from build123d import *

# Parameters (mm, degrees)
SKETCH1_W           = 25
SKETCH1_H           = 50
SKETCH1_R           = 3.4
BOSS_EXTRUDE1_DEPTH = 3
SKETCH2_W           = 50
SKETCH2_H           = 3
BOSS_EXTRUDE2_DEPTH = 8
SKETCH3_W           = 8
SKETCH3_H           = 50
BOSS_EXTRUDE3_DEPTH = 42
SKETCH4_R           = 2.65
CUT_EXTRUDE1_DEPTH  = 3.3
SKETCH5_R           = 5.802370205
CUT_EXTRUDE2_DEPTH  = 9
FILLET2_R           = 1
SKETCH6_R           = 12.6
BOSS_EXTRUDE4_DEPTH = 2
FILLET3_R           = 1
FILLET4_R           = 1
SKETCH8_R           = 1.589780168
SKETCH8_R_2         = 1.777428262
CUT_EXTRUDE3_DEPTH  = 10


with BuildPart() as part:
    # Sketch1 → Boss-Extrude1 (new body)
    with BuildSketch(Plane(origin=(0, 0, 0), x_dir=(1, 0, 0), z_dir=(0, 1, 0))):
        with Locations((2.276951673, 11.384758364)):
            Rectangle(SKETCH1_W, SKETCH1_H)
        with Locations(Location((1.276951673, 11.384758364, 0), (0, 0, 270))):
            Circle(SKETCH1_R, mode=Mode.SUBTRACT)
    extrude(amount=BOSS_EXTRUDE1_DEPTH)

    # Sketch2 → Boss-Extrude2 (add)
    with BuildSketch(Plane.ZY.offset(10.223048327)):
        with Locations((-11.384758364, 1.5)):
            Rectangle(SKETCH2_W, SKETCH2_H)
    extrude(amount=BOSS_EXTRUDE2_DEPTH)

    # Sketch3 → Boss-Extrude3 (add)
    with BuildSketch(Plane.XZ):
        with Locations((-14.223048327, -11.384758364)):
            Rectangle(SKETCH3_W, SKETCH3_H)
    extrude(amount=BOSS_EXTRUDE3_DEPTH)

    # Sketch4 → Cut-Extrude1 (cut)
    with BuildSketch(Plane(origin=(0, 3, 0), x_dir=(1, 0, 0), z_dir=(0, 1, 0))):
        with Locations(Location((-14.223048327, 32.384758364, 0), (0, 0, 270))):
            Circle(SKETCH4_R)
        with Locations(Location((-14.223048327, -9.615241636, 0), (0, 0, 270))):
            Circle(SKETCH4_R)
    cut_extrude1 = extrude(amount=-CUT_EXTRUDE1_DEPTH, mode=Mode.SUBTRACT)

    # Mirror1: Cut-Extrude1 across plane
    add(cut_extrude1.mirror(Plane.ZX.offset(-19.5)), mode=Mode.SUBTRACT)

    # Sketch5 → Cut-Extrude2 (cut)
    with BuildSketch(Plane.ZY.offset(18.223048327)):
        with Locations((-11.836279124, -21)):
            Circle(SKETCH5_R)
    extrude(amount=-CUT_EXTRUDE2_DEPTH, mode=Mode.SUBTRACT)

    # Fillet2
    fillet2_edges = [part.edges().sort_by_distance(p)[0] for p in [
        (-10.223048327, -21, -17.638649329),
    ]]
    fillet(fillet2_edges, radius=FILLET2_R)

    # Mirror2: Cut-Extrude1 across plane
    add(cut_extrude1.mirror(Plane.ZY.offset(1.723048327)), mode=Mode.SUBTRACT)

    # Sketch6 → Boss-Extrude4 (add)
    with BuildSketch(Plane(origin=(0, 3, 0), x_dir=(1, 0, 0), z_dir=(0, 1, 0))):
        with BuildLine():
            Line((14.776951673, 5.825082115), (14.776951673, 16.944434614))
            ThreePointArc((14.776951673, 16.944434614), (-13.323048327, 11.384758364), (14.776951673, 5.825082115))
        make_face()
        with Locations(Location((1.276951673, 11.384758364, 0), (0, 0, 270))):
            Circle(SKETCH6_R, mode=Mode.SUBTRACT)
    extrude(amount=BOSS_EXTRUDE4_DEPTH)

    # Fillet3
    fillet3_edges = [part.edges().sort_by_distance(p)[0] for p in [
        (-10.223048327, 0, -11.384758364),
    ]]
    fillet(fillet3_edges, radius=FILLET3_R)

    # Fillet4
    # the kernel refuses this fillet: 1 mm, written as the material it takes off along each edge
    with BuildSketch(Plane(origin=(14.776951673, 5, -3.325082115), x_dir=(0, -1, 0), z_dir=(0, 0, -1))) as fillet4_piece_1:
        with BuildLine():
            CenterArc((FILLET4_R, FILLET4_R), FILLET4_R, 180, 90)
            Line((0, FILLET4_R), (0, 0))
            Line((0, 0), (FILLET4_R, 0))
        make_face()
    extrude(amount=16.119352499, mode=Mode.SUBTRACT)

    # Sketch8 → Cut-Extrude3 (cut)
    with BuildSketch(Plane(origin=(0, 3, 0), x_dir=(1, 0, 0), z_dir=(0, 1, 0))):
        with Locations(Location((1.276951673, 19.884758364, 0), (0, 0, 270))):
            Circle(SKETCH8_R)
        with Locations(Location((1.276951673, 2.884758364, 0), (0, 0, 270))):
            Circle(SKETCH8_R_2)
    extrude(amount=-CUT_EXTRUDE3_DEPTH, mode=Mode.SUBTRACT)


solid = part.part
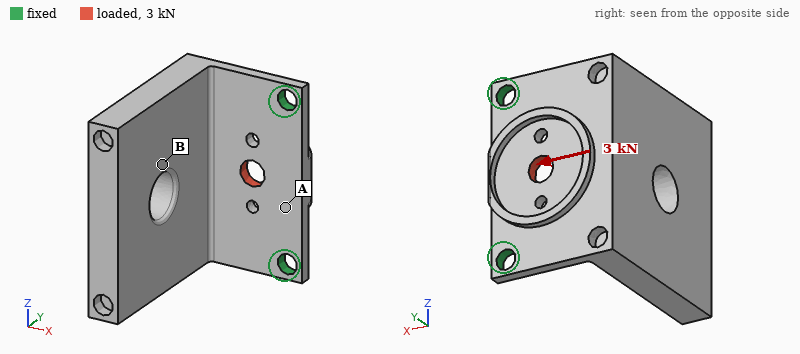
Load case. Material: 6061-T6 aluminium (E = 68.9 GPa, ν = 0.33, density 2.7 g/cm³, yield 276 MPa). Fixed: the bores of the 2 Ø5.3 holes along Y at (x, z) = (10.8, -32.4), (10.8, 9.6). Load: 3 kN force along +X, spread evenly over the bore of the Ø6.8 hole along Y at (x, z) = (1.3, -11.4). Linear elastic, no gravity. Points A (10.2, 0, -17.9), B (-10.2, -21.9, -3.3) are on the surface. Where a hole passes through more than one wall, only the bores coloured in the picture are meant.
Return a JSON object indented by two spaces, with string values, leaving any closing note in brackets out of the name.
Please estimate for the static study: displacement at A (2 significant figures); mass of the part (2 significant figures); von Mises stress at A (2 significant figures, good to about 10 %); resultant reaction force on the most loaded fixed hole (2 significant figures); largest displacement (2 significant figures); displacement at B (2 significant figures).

{
  "displacement at A": "16 µm",
  "mass of the part": "56 g",
  "von Mises stress at A": "29 MPa",
  "resultant reaction force on the most loaded fixed hole": "1.6 kN",
  "largest displacement": "31 µm",
  "displacement at B": "21 µm"
}
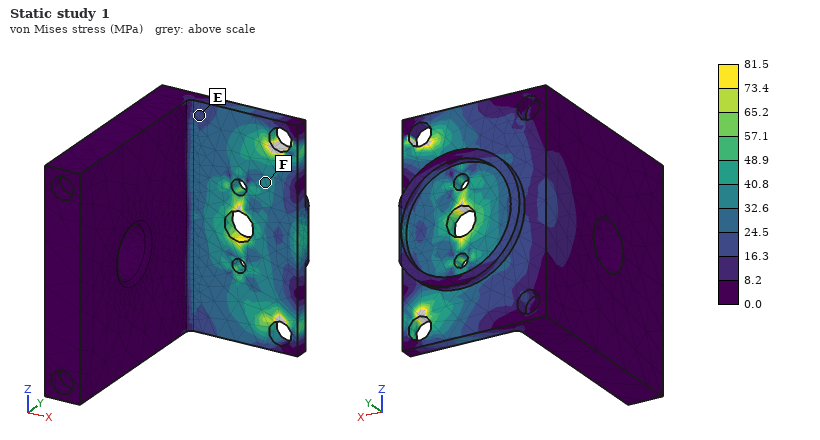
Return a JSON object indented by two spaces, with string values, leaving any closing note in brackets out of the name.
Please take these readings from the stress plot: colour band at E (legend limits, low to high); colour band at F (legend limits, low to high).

{
  "colour band at E": "16.3 to 24.5 MPa",
  "colour band at F": "32.6 to 40.8 MPa"
}
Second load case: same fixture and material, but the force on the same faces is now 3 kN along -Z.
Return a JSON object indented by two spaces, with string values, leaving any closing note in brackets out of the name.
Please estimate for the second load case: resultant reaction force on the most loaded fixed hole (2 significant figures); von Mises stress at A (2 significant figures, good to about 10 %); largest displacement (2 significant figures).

{
  "resultant reaction force on the most loaded fixed hole": "1.6 kN",
  "von Mises stress at A": "25 MPa",
  "largest displacement": "18 µm"
}
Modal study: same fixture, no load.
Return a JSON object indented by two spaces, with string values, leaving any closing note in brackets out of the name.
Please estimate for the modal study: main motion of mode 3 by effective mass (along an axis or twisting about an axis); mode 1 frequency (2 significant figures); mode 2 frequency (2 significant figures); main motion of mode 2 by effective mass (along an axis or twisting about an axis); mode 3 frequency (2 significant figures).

{
  "main motion of mode 3 by effective mass": "along Y",
  "mode 1 frequency": "490 Hz",
  "mode 2 frequency": "1300 Hz",
  "main motion of mode 2 by effective mass": "along Z",
  "mode 3 frequency": "2200 Hz"
}
